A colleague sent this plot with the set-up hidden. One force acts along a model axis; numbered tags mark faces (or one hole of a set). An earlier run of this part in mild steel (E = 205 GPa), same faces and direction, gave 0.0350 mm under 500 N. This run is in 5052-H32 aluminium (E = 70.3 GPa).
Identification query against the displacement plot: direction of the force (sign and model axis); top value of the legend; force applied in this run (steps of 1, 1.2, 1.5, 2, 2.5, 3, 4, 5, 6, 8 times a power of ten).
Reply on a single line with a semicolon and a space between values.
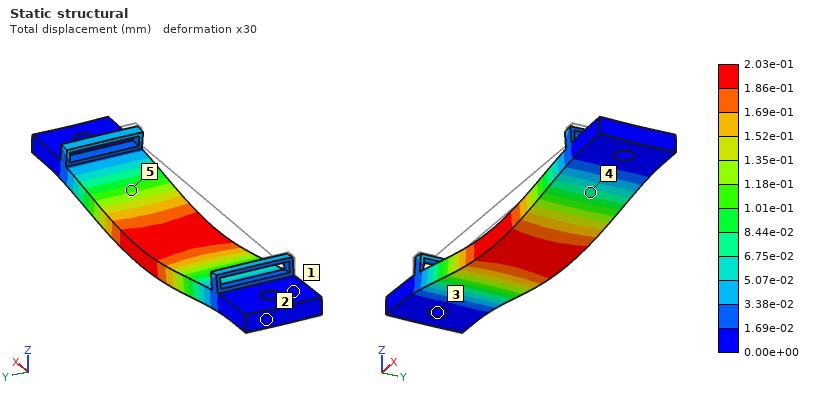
-Z; 2.03e-01 mm; 1 kN
